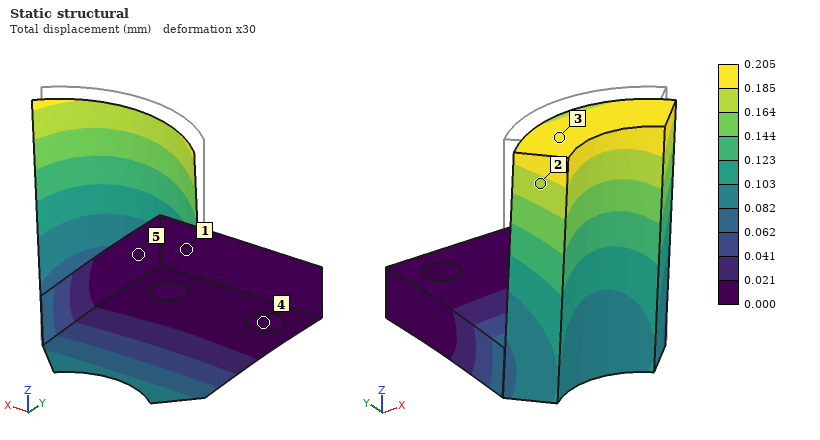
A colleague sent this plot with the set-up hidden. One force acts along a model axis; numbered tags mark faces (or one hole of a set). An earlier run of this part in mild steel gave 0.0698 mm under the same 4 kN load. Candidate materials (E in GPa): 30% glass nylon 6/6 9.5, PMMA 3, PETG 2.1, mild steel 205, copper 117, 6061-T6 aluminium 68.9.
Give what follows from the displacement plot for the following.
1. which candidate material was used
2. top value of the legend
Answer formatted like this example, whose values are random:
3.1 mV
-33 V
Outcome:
6061-T6 aluminium
0.205 mm
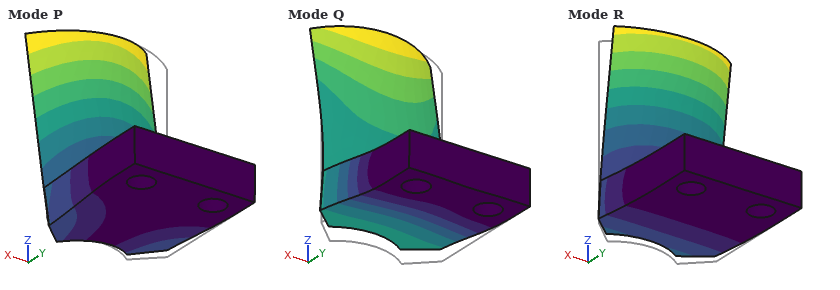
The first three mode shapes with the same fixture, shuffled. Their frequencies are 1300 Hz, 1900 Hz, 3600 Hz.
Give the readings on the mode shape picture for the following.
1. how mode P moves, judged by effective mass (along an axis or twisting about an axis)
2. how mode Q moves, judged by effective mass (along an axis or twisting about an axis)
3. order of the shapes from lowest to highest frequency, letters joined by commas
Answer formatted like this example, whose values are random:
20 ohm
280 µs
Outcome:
along X
along Z
R, P, Q
